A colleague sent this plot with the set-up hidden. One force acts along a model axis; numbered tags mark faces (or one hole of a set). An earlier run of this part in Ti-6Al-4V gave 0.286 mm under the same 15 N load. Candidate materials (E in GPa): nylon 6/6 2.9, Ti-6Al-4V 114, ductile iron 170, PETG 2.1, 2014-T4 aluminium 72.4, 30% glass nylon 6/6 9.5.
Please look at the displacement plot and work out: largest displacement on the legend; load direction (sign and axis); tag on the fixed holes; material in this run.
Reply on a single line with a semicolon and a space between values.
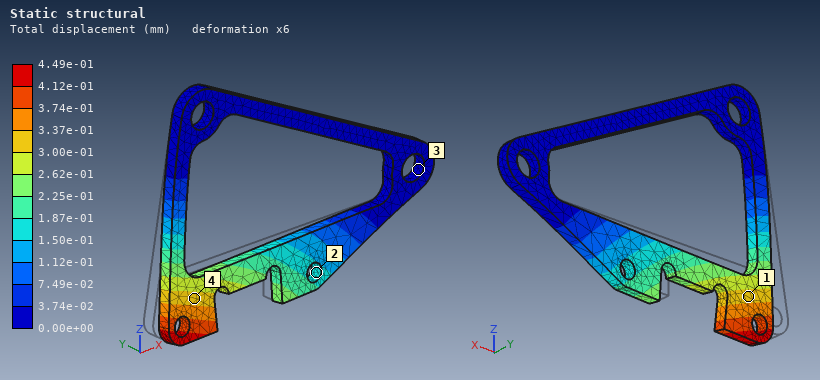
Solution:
4.49e-01 mm; -Y; 3; 2014-T4 aluminium
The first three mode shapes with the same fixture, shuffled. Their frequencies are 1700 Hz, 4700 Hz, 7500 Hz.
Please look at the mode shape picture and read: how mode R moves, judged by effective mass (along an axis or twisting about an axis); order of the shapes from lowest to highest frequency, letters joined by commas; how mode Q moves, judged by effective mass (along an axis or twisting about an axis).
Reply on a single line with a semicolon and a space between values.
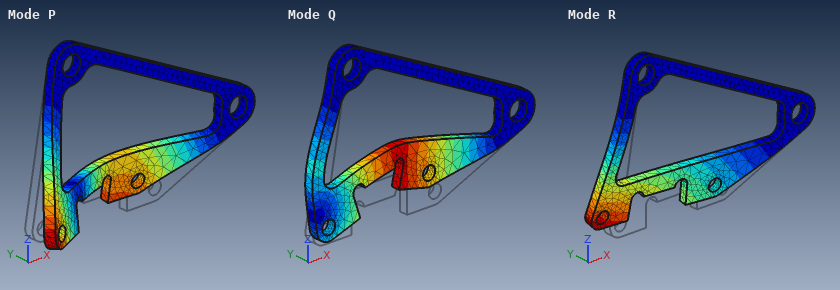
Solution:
along Y; R, P, Q; along Z
